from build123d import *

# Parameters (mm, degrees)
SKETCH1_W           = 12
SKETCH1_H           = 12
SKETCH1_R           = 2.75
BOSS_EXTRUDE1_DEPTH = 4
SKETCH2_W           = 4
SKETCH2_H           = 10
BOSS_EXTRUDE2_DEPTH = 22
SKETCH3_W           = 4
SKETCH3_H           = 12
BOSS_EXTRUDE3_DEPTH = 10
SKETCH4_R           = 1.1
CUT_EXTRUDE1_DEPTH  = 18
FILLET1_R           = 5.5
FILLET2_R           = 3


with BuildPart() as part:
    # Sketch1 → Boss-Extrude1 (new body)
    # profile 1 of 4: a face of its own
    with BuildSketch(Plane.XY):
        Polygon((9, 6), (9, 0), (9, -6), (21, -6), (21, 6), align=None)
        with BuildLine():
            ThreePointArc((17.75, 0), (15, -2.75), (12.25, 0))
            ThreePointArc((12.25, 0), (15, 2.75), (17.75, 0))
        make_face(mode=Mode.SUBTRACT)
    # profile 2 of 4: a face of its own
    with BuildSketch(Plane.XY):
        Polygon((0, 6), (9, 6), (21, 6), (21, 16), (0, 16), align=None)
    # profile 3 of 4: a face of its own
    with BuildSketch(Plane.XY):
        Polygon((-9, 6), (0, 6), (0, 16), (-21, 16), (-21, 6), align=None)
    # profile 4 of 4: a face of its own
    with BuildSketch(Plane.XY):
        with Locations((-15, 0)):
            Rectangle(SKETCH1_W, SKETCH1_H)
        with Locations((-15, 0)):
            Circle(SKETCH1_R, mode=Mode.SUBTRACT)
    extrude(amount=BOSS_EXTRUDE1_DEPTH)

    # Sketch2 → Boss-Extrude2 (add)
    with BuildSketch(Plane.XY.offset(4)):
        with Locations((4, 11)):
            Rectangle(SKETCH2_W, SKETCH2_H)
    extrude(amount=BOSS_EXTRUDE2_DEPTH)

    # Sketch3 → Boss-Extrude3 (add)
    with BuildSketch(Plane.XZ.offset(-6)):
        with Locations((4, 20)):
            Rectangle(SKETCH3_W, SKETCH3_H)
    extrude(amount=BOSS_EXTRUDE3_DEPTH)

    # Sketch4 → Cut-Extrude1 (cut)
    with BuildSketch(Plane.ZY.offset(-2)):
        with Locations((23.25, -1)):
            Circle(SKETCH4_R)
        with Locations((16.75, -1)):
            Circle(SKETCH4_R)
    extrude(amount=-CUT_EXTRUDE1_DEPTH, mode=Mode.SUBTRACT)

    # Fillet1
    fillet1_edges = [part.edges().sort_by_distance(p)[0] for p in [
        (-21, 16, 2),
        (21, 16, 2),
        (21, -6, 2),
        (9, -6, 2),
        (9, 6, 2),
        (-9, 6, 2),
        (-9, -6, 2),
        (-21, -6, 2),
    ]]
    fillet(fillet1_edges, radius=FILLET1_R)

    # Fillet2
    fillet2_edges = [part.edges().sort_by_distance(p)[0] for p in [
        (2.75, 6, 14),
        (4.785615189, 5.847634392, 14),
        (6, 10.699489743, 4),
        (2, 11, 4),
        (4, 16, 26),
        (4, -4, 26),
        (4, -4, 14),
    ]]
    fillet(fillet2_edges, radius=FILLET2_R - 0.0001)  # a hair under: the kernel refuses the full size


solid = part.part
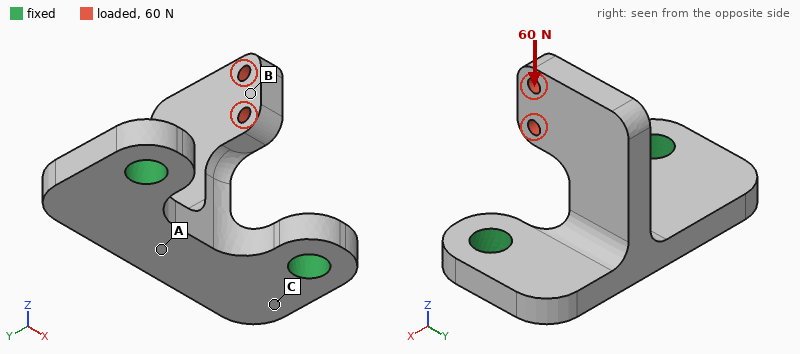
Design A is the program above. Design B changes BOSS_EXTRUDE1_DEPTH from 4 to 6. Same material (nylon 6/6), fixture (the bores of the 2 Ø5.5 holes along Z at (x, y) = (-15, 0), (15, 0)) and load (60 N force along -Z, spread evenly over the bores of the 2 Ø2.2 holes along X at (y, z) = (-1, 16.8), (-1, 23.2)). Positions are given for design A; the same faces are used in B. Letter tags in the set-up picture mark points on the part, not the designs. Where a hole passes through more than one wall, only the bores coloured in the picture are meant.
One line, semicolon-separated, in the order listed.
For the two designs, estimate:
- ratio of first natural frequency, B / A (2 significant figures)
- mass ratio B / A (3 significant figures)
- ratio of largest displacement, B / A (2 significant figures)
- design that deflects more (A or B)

1.4; 1.30; 0.54; A
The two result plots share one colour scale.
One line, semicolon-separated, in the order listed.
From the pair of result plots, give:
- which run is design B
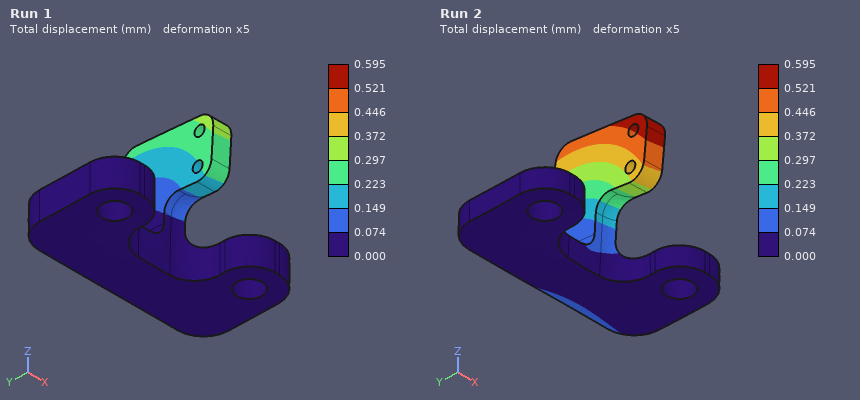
Run 1
